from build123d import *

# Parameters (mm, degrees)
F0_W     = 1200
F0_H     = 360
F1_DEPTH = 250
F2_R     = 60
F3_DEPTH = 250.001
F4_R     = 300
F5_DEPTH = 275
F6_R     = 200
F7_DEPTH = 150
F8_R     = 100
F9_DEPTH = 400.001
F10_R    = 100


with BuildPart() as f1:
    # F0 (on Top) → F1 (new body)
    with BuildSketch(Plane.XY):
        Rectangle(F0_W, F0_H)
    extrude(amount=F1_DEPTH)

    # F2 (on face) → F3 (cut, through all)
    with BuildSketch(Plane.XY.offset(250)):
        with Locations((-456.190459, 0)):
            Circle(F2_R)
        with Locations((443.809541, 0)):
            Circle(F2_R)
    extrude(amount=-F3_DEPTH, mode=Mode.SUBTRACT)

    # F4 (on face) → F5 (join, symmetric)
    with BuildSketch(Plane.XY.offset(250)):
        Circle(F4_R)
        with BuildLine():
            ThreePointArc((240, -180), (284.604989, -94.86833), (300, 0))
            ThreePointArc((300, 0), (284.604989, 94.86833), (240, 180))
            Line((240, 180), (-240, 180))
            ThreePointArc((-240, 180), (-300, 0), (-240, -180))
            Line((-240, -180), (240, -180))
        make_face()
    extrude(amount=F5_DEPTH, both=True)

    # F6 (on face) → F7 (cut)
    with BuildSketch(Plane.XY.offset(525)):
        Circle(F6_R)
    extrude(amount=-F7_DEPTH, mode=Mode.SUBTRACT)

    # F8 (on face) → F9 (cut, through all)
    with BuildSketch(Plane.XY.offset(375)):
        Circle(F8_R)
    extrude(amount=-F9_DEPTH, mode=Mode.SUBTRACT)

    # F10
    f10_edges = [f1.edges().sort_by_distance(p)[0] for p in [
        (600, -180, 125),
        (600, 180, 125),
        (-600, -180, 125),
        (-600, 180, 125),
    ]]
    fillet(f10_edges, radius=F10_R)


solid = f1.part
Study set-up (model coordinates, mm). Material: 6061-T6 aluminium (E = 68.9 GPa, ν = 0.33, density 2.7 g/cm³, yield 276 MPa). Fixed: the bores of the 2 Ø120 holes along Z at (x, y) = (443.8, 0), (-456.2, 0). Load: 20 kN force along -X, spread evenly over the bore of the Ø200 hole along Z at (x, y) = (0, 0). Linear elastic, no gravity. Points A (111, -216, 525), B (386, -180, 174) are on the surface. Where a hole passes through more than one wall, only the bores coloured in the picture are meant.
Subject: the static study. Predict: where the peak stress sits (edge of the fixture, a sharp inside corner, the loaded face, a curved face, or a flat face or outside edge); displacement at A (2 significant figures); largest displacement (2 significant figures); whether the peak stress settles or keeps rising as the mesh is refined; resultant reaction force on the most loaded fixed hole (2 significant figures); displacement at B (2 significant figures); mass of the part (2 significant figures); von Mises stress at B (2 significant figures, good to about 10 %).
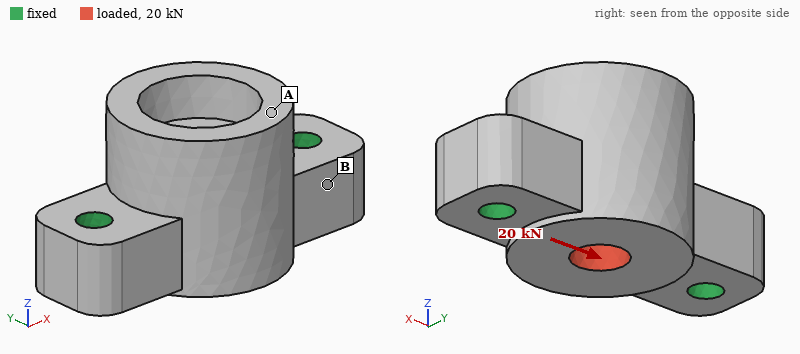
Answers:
edge of the fixture
0.60 µm
0.74 µm
keeps rising
10 kN
0.25 µm
470 kg
0.053 MPa
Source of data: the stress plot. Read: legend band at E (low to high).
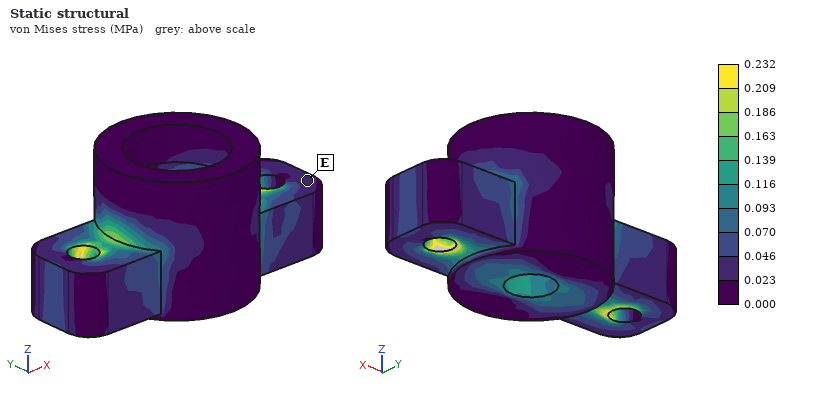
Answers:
0.023 to 0.046 MPa
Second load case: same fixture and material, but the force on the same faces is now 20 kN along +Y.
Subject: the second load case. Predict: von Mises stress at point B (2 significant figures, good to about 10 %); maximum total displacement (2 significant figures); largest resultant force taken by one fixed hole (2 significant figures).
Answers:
0.15 MPa
3.4 µm
10 kN
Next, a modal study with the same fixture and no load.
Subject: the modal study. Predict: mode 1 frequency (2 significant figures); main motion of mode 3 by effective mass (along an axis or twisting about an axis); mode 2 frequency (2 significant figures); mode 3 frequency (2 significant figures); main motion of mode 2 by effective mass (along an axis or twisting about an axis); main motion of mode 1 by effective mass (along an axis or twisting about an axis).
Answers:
550 Hz
along Y
890 Hz
1100 Hz
along Z
along Y
